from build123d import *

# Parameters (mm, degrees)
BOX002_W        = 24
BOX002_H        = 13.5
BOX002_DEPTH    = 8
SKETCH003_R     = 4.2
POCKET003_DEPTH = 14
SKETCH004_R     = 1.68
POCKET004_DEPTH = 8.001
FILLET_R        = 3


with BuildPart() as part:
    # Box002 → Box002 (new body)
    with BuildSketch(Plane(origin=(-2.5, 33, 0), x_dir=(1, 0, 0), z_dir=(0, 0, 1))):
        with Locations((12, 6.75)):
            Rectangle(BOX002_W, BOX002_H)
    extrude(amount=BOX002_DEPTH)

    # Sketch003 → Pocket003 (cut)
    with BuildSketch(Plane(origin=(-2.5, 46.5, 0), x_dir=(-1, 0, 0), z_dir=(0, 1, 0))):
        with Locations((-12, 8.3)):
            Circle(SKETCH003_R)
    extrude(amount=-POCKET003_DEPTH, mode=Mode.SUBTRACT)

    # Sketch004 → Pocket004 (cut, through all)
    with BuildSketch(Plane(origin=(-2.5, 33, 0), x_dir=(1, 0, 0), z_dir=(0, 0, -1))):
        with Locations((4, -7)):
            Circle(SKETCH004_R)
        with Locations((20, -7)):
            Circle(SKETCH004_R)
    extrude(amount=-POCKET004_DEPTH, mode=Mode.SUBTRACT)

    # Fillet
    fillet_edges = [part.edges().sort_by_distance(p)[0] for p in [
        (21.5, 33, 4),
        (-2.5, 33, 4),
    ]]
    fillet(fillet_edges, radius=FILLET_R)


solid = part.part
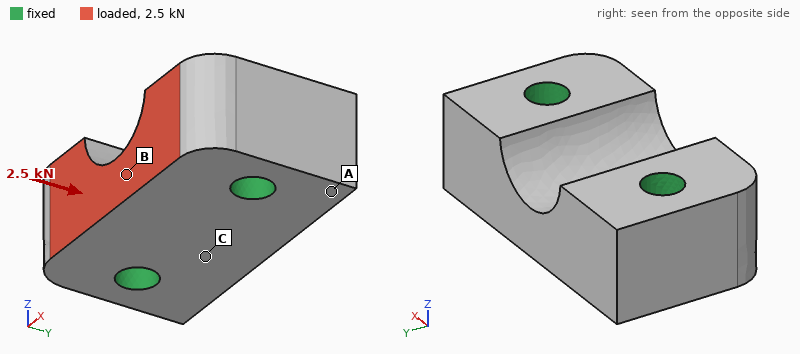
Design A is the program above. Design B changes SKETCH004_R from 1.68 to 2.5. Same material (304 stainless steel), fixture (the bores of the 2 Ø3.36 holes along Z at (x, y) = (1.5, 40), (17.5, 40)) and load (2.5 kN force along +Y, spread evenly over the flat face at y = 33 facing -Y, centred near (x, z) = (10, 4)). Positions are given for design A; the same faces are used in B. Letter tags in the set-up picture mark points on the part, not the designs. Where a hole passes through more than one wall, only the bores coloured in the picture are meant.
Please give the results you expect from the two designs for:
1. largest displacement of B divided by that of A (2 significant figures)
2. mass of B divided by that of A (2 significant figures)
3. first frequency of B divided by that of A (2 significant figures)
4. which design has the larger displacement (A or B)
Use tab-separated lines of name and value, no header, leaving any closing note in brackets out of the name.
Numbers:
largest displacement of B divided by that of A	0.80
mass of B divided by that of A	0.92
first frequency of B divided by that of A	1.3
which design has the larger displacement	A
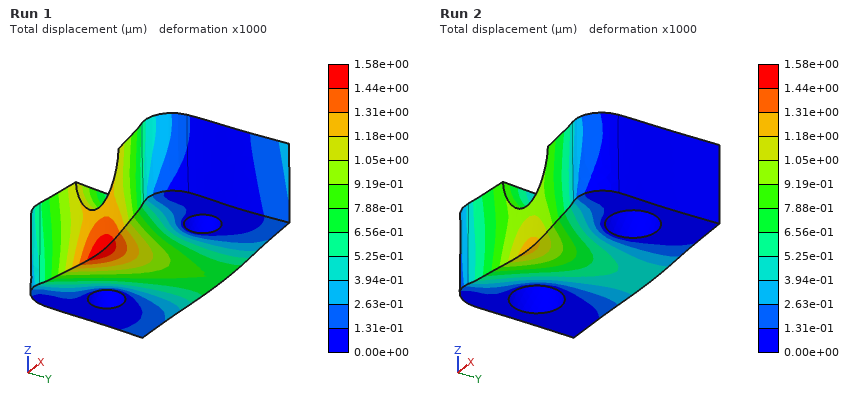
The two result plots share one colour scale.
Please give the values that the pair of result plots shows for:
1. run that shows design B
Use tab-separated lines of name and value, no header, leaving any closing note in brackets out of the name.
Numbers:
run that shows design B	Run 2
